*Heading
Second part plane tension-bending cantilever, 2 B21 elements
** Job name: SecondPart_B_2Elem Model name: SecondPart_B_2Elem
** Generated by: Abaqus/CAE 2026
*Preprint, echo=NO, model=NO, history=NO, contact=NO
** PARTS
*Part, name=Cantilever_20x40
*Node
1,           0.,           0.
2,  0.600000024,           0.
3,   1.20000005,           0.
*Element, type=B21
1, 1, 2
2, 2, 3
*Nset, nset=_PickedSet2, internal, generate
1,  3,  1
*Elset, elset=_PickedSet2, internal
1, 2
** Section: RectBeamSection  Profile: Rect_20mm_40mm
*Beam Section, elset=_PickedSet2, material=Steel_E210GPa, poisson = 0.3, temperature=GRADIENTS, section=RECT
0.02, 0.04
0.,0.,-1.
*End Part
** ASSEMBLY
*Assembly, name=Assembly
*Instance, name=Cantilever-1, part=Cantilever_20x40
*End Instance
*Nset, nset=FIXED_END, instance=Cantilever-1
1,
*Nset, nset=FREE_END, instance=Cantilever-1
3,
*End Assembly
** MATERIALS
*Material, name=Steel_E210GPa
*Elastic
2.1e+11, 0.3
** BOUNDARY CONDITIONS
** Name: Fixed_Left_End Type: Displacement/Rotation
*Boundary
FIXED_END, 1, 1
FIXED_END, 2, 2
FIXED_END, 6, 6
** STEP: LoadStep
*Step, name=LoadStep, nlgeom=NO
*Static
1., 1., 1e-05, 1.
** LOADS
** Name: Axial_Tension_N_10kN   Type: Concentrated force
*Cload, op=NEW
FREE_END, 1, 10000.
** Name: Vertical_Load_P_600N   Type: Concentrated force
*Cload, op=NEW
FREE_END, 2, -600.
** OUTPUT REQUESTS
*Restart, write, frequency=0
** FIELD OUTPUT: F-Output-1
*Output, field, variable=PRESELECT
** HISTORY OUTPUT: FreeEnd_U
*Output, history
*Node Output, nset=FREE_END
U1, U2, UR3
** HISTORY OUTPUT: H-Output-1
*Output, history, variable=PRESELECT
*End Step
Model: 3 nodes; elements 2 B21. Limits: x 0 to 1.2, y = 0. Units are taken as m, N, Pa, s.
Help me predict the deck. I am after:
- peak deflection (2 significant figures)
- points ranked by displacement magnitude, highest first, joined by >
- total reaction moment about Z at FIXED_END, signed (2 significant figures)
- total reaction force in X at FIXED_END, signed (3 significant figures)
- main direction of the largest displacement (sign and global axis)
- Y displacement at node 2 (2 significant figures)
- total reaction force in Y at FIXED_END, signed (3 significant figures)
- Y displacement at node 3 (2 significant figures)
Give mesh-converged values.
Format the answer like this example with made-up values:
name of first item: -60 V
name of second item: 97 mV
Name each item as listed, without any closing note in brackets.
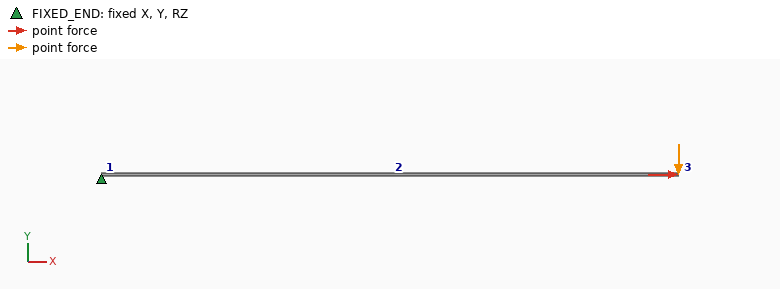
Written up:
peak deflection: 0.015 m
points ranked by displacement magnitude, highest first, joined by >: node 3 > node 2 > node 1
total reaction moment about Z at FIXED_END, signed: 720 N·m
total reaction force in X at FIXED_END, signed: -10000 N
main direction of the largest displacement: -Y
Y displacement at node 2: -0.0048 m
total reaction force in Y at FIXED_END, signed: 600 N
Y displacement at node 3: -0.015 m
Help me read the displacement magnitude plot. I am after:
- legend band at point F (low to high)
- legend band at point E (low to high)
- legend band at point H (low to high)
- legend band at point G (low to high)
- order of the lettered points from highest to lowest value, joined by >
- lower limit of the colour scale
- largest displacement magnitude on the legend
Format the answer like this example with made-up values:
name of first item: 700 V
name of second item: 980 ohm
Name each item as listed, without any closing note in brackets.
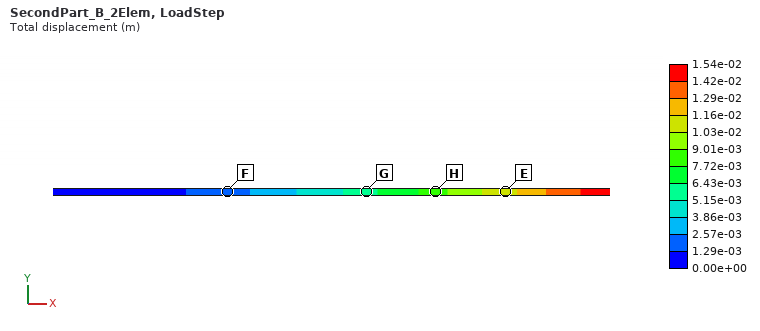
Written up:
legend band at point F: 1.29e-03 to 2.57e-03 m
legend band at point E: 1.03e-02 to 1.16e-02 m
legend band at point H: 7.72e-03 to 9.01e-03 m
legend band at point G: 5.15e-03 to 6.43e-03 m
order of the lettered points from highest to lowest value, joined by >: E > H > G > F
lower limit of the colour scale: 0.00e+00 m
largest displacement magnitude on the legend: 1.54e-02 m
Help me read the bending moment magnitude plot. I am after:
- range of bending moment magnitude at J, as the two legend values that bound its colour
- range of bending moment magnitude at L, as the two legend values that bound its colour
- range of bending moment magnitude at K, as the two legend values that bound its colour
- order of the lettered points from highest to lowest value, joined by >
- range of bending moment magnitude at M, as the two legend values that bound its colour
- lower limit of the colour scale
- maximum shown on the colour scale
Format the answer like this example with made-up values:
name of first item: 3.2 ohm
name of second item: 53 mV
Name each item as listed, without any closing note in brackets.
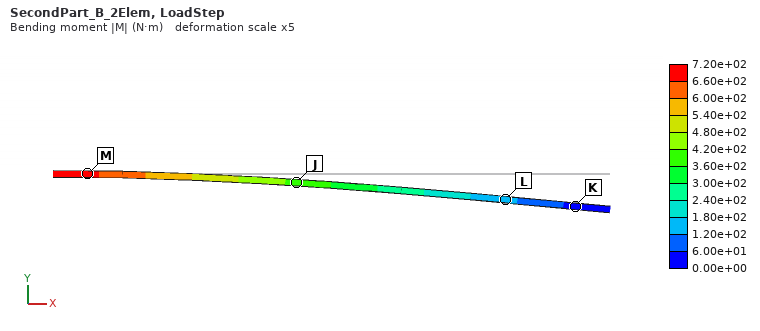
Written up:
range of bending moment magnitude at J, as the two legend values that bound its colour: 3.60e+02 to 4.20e+02 N·m
range of bending moment magnitude at L, as the two legend values that bound its colour: 1.20e+02 to 1.80e+02 N·m
range of bending moment magnitude at K, as the two legend values that bound its colour: 0.00e+00 to 6.00e+01 N·m
order of the lettered points from highest to lowest value, joined by >: M > J > L > K
range of bending moment magnitude at M, as the two legend values that bound its colour: 6.60e+02 to 7.20e+02 N·m
lower limit of the colour scale: 0.00e+00 N·m
maximum shown on the colour scale: 7.20e+02 N·m
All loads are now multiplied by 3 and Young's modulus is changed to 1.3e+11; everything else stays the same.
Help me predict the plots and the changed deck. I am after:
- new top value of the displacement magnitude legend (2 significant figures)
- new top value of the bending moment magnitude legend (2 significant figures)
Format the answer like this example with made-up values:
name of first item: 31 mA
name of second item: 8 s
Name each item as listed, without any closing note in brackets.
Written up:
new top value of the displacement magnitude legend: 0.075 m
new top value of the bending moment magnitude legend: 2200 N·m
